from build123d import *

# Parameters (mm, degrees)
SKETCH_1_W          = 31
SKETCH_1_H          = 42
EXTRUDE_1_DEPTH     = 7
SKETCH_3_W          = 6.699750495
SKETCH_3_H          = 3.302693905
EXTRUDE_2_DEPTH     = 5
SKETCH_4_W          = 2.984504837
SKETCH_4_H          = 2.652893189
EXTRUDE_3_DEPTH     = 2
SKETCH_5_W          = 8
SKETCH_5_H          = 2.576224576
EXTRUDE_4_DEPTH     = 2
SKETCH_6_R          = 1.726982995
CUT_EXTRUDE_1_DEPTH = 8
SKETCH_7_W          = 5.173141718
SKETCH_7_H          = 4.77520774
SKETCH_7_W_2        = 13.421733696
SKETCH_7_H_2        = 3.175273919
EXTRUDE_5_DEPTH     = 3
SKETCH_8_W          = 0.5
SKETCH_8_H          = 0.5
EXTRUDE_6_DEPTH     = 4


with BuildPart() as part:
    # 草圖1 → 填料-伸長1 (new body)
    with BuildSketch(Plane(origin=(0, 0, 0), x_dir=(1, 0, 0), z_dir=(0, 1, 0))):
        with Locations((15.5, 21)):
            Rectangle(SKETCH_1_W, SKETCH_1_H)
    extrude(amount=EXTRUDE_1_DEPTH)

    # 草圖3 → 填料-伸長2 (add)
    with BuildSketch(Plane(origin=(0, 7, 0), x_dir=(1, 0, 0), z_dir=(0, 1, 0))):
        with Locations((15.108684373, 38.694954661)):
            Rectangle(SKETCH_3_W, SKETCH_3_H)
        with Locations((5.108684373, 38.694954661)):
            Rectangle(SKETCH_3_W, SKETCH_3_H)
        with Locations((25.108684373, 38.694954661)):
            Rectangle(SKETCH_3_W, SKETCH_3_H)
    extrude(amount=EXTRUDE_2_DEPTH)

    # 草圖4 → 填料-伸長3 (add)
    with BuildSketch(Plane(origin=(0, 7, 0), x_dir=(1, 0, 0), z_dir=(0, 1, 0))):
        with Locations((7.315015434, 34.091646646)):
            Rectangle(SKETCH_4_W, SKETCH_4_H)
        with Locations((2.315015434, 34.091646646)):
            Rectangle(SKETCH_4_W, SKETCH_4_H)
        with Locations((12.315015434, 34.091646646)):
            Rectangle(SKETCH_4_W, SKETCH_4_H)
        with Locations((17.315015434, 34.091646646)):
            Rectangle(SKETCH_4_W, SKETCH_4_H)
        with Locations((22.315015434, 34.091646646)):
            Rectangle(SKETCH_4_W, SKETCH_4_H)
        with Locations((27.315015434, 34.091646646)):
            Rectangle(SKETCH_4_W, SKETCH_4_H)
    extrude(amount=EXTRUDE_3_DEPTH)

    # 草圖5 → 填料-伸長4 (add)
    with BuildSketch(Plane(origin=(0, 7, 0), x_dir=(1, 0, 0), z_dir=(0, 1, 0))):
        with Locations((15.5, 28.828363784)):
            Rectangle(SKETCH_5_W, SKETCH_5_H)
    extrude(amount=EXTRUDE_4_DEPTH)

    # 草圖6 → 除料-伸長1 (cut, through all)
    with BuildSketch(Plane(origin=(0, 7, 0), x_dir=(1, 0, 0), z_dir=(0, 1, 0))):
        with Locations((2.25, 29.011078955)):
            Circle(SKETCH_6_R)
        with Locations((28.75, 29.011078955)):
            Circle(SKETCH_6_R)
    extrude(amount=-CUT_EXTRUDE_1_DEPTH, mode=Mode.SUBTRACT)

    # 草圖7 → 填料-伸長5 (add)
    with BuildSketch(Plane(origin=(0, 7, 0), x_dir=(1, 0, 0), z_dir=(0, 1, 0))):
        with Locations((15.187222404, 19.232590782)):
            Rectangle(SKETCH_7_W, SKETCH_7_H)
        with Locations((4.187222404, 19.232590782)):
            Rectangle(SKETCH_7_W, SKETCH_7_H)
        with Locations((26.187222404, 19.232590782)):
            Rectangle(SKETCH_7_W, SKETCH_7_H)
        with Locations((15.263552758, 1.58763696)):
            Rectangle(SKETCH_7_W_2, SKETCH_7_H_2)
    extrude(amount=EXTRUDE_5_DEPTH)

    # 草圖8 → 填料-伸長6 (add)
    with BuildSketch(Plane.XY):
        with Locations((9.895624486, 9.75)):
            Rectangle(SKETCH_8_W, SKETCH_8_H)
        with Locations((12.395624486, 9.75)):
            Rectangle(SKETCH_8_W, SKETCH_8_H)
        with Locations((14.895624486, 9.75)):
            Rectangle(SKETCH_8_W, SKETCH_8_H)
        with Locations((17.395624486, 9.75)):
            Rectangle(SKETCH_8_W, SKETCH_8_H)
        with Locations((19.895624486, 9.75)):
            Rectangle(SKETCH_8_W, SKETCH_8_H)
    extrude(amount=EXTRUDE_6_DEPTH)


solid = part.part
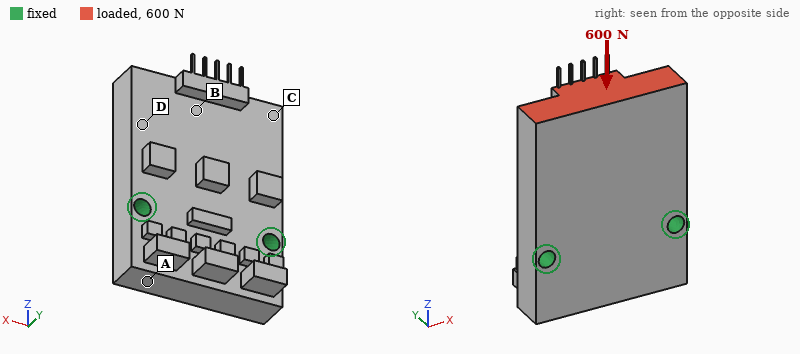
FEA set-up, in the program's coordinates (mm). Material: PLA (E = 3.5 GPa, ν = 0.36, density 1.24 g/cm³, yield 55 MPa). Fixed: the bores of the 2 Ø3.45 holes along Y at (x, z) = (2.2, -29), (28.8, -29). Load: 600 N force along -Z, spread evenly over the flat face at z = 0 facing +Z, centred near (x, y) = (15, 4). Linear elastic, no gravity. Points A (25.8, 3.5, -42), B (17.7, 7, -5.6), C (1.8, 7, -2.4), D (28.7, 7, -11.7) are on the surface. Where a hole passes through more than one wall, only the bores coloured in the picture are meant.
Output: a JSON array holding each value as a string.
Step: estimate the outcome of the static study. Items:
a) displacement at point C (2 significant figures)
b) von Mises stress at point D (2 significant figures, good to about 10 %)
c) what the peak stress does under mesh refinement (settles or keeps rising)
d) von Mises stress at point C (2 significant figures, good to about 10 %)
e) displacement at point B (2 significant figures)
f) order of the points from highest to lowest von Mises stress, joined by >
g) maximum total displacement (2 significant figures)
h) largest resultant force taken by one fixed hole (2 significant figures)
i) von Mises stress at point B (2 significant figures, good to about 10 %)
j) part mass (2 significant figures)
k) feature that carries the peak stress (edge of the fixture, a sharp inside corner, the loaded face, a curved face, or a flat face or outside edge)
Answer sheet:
["0.063 mm", "4.2 MPa", "keeps rising", "2.5 MPa", "0.058 mm", "B > D > C > A", "0.12 mm", "300 N", "6.1 MPa", "12 g", "edge of the fixture"]
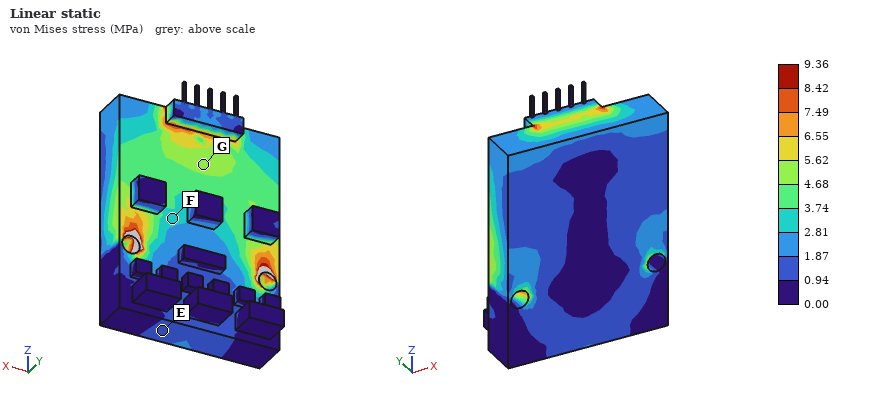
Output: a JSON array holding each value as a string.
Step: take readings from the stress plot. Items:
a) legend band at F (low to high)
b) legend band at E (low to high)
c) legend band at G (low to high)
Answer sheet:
["2.81 to 3.74 MPa", "0.94 to 1.87 MPa", "4.68 to 5.62 MPa"]
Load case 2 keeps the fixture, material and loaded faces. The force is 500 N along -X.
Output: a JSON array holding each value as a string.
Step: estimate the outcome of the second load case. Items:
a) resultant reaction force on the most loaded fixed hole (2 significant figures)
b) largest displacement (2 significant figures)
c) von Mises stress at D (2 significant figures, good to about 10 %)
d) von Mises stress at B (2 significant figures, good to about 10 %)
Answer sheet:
["590 N", "0.15 mm", "5.0 MPa", "7.5 MPa"]
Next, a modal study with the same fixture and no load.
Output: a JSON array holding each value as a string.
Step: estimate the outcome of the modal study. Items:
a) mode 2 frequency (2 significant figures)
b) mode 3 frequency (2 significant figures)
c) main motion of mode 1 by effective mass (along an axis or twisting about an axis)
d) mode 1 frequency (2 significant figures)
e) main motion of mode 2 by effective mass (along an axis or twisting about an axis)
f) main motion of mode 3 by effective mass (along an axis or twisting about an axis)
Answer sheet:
["4600 Hz", "6100 Hz", "along Y", "1900 Hz", "twisting about Z", "along X"]
